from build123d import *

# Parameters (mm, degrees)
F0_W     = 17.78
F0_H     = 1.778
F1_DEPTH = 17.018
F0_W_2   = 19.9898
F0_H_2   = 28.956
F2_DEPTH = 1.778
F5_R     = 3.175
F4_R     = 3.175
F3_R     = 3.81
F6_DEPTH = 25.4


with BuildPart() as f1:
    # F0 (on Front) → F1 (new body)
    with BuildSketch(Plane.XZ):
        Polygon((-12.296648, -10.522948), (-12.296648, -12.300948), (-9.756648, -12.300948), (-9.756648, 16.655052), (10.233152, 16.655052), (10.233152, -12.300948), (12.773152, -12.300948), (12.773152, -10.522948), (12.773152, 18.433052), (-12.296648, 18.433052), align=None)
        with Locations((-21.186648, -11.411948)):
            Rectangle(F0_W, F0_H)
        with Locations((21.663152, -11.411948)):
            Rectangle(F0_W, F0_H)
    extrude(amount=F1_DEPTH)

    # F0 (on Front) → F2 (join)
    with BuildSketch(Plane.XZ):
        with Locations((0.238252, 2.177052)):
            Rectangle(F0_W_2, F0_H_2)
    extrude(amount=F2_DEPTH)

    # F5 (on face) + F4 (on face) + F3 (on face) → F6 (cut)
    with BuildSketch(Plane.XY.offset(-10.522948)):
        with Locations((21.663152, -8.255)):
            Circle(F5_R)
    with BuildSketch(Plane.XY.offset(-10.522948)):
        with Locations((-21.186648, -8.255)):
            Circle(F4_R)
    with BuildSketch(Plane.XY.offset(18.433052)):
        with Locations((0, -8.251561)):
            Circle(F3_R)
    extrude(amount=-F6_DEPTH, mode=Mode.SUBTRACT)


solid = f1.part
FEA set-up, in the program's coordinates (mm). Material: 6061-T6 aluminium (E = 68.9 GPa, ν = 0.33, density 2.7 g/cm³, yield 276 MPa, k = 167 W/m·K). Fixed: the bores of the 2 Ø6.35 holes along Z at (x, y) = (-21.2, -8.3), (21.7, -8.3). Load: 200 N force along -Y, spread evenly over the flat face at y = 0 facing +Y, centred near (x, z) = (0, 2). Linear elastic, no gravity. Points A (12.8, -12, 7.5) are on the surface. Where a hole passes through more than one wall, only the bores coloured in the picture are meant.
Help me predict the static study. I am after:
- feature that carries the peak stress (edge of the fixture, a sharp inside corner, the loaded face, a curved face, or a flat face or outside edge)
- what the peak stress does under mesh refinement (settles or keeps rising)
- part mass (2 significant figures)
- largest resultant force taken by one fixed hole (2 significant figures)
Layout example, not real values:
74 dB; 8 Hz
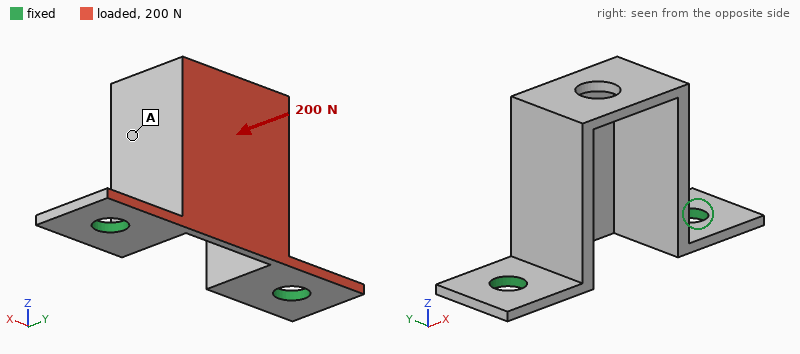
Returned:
edge of the fixture; keeps rising; 14 g; 100 N
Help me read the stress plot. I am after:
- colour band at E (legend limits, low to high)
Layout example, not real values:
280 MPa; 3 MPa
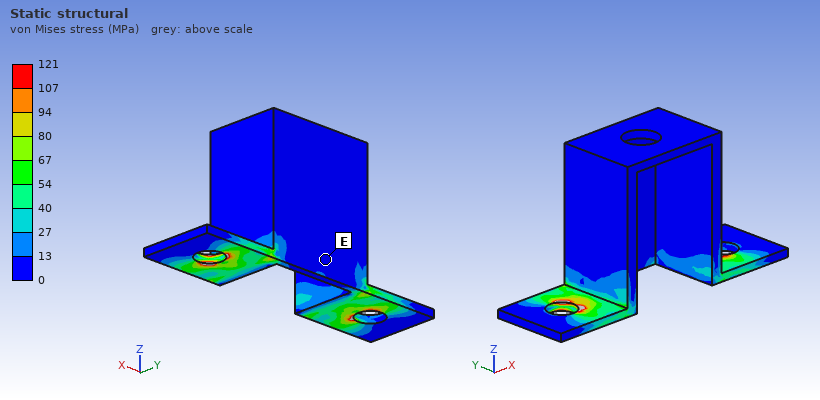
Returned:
0 to 13 MPa
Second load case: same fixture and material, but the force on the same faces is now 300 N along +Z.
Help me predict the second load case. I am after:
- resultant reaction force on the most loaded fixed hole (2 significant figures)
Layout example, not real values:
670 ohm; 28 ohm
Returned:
170 N
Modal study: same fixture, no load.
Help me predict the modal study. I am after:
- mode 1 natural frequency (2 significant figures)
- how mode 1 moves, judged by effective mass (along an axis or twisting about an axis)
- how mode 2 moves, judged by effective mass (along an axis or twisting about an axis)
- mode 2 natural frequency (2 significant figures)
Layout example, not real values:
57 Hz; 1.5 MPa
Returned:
1500 Hz; along Y; along X; 2800 Hz
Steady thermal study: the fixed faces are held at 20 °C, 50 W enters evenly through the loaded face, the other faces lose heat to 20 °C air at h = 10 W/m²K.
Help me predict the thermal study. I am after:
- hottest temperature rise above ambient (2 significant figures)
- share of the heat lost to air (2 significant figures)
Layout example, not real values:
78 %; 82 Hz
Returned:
82 K; 4.7 %
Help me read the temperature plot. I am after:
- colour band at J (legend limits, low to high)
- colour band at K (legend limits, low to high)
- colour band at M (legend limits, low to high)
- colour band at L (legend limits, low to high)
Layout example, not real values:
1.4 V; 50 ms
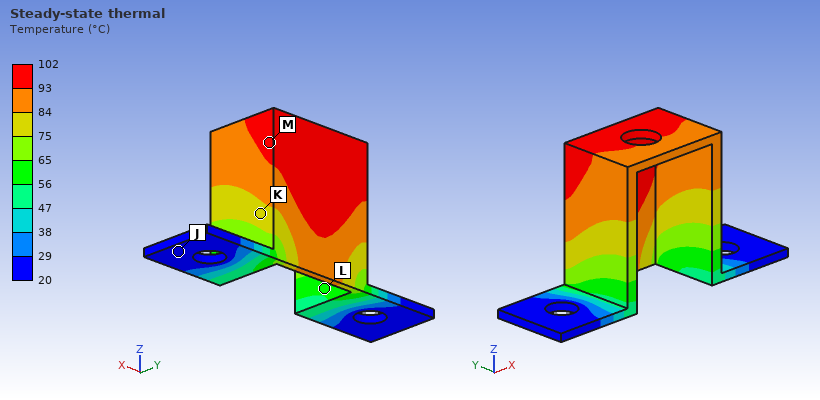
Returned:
20 to 29 °C; 75 to 84 °C; 93 to 102 °C; 56 to 65 °C
